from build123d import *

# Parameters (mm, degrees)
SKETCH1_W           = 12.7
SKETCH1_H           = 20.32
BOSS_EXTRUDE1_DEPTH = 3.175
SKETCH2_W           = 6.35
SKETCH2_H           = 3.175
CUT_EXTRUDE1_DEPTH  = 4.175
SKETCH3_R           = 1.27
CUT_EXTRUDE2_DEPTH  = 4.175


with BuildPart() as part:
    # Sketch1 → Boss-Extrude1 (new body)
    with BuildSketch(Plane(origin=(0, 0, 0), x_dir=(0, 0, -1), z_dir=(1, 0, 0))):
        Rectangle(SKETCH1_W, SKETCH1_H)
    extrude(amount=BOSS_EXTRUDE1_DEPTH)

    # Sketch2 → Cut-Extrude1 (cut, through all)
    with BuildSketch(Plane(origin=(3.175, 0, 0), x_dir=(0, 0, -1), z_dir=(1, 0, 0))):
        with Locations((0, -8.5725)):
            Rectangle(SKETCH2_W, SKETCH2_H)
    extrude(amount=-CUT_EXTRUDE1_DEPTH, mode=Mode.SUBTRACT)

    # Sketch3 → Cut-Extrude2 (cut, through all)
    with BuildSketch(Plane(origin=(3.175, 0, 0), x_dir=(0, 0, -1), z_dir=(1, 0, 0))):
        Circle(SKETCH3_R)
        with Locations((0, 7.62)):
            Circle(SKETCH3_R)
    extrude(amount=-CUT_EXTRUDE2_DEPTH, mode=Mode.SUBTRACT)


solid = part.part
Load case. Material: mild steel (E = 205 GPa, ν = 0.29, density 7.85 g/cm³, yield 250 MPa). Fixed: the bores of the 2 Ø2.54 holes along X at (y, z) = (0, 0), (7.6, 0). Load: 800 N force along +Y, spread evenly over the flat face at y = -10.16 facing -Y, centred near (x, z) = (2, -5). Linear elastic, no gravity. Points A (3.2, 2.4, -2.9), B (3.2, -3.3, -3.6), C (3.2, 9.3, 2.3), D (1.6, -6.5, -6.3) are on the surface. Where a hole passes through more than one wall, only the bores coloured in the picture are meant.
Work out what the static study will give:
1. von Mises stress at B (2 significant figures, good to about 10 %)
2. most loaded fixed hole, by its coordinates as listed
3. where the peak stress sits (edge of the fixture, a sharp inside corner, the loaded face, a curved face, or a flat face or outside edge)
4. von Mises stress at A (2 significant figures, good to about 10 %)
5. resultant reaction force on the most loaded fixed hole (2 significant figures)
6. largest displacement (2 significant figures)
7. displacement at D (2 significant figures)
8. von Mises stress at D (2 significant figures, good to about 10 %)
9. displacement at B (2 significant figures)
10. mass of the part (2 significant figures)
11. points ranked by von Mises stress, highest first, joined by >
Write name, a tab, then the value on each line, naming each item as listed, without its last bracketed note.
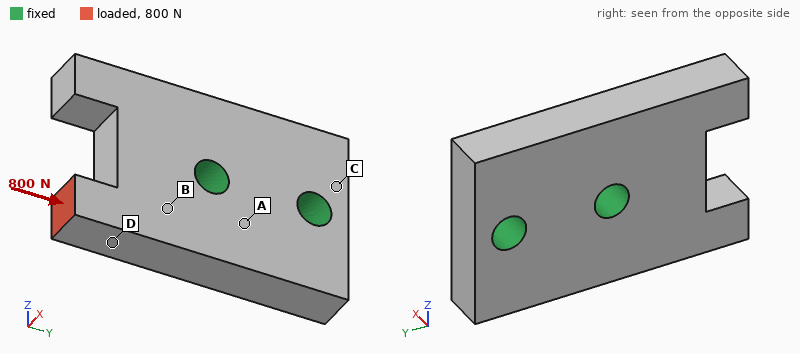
von Mises stress at B	49 MPa
most loaded fixed hole, by its coordinates as listed	(0, 0)
where the peak stress sits	edge of the fixture
von Mises stress at A	37 MPa
resultant reaction force on the most loaded fixed hole	690 N
largest displacement	7.9 µm
displacement at D	5.2 µm
von Mises stress at D	90 MPa
displacement at B	1.9 µm
mass of the part	5.7 g
points ranked by von Mises stress, highest first, joined by >	D > B > A > C
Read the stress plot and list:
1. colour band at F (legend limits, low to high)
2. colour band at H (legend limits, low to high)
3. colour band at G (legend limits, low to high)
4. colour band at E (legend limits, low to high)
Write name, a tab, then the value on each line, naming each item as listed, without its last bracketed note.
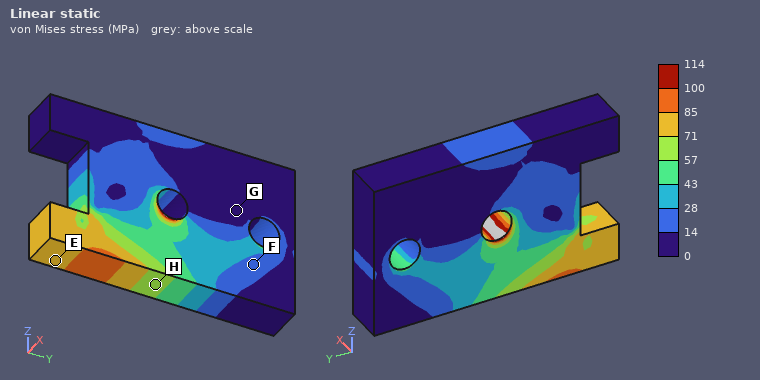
colour band at F	14 to 28 MPa
colour band at H	57 to 71 MPa
colour band at G	0 to 14 MPa
colour band at E	71 to 85 MPa
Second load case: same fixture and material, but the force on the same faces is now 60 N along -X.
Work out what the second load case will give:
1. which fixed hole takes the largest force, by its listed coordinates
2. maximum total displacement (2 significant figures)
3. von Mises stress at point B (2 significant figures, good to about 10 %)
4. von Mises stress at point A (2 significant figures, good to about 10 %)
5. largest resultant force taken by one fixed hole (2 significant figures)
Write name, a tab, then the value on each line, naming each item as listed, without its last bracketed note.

which fixed hole takes the largest force, by its listed coordinates	(0, 0)
maximum total displacement	7.5 µm
von Mises stress at point B	32 MPa
von Mises stress at point A	10 MPa
largest resultant force taken by one fixed hole	84 N
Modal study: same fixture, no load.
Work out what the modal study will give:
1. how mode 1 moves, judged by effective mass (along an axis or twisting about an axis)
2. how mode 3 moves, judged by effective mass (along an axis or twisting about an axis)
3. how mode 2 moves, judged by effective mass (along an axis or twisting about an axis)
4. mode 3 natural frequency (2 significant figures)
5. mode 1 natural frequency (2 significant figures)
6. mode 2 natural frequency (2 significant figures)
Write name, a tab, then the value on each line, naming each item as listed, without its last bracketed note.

how mode 1 moves, judged by effective mass	along X
how mode 3 moves, judged by effective mass	along Z
how mode 2 moves, judged by effective mass	twisting about Y
mode 3 natural frequency	46 kHz
mode 1 natural frequency	28 kHz
mode 2 natural frequency	32 kHz
